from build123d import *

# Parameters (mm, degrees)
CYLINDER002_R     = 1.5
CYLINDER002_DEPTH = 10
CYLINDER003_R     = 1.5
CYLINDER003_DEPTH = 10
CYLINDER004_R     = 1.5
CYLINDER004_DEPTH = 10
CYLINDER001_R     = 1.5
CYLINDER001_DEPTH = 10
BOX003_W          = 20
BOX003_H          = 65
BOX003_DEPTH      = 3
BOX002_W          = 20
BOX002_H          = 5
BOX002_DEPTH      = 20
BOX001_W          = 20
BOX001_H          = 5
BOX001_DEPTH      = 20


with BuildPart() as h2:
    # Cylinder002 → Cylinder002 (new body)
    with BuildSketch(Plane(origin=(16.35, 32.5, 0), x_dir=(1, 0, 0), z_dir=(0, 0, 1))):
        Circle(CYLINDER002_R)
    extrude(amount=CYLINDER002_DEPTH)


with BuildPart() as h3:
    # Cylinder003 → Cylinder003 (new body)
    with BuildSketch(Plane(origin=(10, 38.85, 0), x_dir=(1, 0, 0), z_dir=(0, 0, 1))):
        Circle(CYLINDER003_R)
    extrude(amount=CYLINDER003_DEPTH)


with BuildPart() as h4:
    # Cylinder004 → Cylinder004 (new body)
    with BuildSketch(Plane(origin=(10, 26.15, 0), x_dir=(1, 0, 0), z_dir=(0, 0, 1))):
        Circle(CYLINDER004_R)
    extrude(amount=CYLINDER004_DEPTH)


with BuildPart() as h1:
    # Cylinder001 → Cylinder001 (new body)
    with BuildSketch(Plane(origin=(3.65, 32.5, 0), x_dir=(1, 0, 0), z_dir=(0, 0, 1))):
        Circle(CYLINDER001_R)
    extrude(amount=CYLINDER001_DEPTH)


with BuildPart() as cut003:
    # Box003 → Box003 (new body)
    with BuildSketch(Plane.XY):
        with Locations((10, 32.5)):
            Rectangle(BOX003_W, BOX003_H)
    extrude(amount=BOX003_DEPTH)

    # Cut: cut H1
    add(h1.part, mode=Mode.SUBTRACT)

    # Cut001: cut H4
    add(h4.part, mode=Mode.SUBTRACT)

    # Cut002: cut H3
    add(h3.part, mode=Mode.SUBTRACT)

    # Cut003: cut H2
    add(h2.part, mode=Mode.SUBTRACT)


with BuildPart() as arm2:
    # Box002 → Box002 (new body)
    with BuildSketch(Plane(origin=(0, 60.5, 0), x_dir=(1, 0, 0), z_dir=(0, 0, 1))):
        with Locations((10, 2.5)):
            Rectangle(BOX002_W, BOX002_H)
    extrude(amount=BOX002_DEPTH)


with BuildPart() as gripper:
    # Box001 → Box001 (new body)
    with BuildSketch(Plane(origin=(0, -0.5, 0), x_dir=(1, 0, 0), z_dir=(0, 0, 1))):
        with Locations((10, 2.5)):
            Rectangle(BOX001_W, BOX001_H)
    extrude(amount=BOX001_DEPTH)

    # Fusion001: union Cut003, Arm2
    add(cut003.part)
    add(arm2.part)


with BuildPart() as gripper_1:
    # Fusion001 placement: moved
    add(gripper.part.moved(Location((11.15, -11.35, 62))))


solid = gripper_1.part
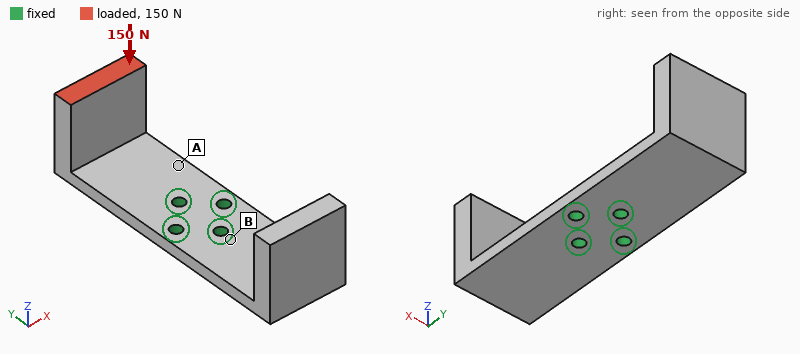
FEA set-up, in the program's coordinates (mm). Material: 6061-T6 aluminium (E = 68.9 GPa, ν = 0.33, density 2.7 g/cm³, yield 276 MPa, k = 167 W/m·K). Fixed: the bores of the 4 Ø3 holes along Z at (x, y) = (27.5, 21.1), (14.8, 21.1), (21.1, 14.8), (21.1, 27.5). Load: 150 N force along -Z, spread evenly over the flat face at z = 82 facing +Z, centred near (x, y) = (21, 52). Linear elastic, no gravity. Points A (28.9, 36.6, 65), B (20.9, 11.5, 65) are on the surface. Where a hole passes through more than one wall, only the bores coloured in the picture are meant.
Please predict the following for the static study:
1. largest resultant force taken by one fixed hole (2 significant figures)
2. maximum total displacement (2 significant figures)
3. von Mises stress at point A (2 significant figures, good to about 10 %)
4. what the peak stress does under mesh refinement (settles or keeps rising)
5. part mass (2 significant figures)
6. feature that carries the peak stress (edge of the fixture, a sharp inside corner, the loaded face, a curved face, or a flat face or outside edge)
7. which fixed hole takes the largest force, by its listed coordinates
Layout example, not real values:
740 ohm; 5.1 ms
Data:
390 N; 0.36 mm; 73 MPa; keeps rising; 20 g; edge of the fixture; (21.1, 27.5)
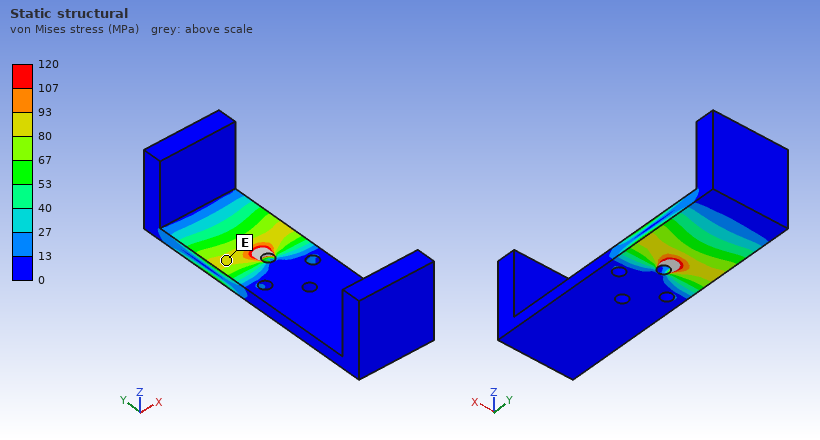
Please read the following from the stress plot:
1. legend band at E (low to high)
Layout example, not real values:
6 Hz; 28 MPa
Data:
80 to 93 MPa
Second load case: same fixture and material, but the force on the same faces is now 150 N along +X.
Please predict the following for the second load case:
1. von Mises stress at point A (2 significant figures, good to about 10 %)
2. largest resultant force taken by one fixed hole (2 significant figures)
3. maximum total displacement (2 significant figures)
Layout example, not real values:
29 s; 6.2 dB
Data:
69 MPa; 210 N; 0.27 mm
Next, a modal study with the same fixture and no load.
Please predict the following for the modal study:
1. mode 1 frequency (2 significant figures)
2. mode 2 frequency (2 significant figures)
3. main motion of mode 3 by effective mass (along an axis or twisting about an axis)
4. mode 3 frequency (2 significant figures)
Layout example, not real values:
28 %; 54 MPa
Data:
1400 Hz; 1400 Hz; twisting about Z; 2600 Hz
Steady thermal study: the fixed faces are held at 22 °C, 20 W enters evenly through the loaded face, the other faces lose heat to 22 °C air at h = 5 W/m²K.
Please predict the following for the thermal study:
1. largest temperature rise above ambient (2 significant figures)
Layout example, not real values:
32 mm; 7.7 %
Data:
69 K
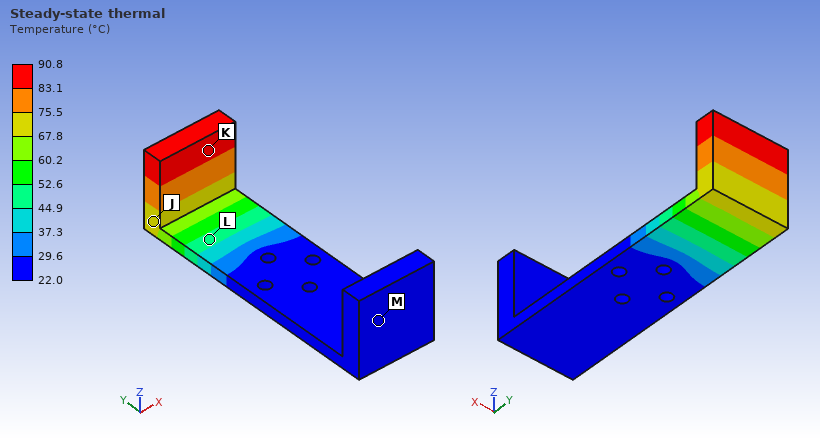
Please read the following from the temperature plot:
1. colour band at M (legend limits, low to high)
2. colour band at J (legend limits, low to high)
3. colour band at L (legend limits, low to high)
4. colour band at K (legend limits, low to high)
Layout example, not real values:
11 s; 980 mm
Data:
22.0 to 29.6 °C; 67.8 to 75.5 °C; 44.9 to 52.6 °C; 83.1 to 90.8 °C
